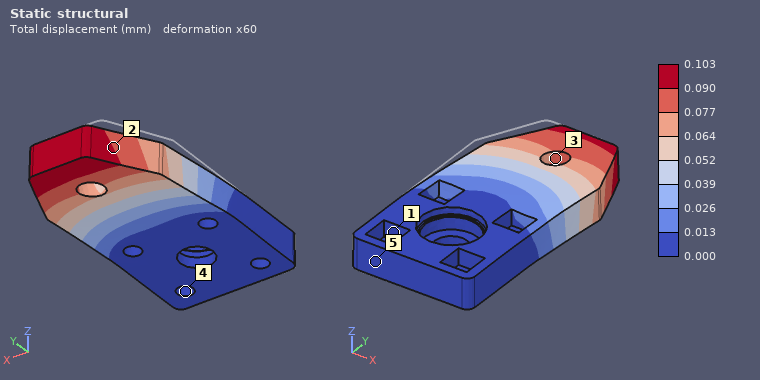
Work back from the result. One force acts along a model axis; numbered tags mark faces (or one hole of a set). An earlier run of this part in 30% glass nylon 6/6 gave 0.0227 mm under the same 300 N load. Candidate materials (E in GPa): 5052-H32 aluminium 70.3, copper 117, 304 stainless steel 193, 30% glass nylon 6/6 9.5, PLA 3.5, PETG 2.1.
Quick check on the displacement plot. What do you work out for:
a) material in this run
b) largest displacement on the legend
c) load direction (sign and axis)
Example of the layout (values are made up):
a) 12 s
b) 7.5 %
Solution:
a) PETG
b) 0.103 mm
c) +X
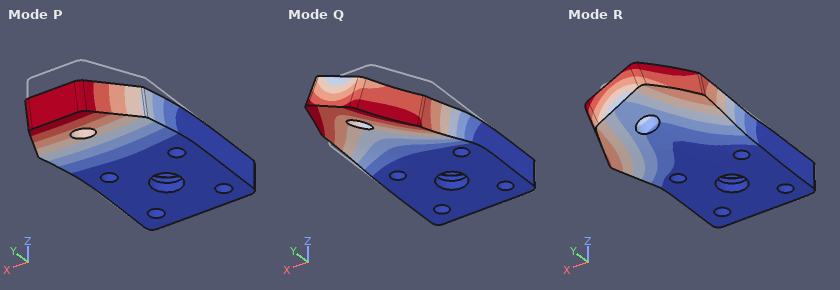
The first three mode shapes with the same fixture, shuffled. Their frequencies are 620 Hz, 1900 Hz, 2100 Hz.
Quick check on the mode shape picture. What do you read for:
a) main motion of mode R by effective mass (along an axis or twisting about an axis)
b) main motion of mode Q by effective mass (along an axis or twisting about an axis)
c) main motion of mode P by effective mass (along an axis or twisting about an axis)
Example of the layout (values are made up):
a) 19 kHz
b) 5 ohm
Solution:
a) along X
b) along X
c) along Z
